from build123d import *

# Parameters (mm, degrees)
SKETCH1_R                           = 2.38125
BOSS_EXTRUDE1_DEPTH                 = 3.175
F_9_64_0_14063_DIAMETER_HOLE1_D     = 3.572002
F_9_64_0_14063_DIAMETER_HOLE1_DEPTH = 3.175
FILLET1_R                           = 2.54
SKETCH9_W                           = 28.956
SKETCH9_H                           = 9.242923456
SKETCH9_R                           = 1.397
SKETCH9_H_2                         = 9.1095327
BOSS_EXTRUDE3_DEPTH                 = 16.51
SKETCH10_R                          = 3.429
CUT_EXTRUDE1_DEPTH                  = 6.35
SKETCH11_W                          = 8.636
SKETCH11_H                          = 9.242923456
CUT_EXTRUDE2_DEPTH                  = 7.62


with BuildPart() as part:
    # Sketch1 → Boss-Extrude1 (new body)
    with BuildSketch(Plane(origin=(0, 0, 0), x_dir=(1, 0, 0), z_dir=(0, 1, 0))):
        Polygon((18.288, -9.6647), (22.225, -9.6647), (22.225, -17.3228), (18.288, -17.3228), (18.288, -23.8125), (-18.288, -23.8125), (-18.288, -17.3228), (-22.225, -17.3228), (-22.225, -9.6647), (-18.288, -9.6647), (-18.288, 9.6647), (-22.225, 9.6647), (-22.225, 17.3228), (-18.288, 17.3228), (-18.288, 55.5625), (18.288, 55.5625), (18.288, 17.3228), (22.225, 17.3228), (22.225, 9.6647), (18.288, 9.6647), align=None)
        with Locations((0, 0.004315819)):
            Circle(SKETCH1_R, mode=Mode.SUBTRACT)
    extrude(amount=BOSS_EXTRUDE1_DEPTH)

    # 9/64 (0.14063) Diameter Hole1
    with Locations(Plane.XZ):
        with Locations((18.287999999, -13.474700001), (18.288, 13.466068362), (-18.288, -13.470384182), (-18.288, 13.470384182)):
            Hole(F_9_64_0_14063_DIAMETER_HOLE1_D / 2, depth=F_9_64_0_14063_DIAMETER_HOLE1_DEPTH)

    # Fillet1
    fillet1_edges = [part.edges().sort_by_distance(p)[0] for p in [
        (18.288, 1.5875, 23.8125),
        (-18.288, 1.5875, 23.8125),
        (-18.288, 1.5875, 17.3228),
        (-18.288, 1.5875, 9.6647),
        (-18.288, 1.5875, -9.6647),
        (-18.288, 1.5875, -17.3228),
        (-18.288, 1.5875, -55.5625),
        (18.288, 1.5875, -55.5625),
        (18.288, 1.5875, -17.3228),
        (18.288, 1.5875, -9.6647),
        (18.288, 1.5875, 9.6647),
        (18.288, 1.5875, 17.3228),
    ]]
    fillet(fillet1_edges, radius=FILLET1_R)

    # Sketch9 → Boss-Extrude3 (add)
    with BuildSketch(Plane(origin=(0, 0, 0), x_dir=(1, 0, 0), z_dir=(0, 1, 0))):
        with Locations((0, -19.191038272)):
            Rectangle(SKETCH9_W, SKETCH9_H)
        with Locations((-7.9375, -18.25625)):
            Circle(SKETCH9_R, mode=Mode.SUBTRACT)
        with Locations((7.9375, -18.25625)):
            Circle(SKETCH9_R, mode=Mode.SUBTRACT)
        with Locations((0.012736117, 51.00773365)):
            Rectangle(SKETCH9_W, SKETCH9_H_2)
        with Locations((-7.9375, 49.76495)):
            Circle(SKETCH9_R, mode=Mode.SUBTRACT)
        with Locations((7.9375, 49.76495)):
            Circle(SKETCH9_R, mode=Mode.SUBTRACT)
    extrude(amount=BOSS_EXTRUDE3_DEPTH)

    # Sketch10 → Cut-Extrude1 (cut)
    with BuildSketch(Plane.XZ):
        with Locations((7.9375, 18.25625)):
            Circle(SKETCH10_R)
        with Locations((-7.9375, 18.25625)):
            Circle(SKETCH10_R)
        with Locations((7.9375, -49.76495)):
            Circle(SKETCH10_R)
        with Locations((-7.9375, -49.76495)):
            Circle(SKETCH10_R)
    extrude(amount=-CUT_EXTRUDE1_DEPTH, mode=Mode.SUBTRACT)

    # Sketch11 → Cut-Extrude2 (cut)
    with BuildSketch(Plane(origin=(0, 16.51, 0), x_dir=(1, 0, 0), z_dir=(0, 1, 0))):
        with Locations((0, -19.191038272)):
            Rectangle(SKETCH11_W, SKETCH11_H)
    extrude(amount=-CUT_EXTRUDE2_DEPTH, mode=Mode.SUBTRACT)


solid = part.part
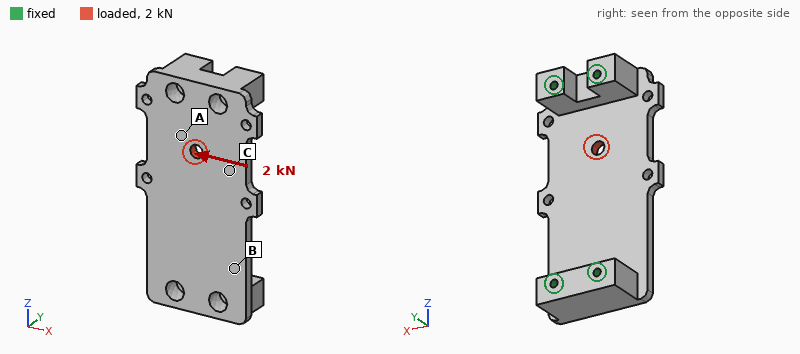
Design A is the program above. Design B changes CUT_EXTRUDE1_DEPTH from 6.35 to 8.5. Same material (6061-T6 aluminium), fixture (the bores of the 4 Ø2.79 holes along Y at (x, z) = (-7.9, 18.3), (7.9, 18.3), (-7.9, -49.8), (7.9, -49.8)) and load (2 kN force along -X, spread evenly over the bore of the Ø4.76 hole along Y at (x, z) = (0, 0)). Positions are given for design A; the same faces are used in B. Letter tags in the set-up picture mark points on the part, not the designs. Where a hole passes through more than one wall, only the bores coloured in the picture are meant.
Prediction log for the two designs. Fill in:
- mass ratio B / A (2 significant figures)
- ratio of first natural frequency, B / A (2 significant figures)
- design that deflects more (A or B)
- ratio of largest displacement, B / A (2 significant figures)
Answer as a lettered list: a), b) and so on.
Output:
a) 0.98
b) 0.99
c) B
d) 1.2
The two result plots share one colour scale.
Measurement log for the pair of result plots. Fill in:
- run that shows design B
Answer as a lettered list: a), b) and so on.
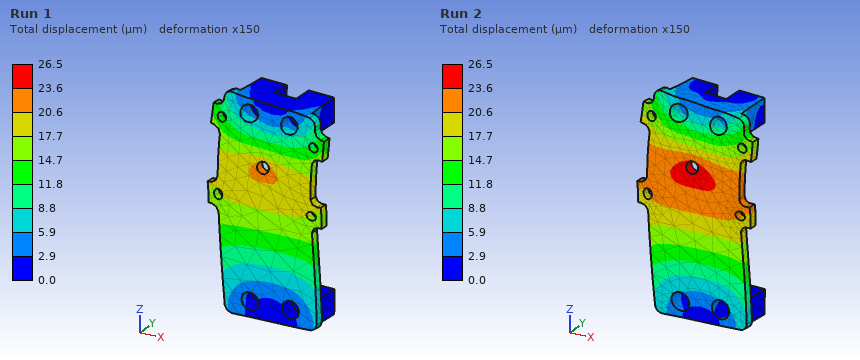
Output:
a) Run 2
